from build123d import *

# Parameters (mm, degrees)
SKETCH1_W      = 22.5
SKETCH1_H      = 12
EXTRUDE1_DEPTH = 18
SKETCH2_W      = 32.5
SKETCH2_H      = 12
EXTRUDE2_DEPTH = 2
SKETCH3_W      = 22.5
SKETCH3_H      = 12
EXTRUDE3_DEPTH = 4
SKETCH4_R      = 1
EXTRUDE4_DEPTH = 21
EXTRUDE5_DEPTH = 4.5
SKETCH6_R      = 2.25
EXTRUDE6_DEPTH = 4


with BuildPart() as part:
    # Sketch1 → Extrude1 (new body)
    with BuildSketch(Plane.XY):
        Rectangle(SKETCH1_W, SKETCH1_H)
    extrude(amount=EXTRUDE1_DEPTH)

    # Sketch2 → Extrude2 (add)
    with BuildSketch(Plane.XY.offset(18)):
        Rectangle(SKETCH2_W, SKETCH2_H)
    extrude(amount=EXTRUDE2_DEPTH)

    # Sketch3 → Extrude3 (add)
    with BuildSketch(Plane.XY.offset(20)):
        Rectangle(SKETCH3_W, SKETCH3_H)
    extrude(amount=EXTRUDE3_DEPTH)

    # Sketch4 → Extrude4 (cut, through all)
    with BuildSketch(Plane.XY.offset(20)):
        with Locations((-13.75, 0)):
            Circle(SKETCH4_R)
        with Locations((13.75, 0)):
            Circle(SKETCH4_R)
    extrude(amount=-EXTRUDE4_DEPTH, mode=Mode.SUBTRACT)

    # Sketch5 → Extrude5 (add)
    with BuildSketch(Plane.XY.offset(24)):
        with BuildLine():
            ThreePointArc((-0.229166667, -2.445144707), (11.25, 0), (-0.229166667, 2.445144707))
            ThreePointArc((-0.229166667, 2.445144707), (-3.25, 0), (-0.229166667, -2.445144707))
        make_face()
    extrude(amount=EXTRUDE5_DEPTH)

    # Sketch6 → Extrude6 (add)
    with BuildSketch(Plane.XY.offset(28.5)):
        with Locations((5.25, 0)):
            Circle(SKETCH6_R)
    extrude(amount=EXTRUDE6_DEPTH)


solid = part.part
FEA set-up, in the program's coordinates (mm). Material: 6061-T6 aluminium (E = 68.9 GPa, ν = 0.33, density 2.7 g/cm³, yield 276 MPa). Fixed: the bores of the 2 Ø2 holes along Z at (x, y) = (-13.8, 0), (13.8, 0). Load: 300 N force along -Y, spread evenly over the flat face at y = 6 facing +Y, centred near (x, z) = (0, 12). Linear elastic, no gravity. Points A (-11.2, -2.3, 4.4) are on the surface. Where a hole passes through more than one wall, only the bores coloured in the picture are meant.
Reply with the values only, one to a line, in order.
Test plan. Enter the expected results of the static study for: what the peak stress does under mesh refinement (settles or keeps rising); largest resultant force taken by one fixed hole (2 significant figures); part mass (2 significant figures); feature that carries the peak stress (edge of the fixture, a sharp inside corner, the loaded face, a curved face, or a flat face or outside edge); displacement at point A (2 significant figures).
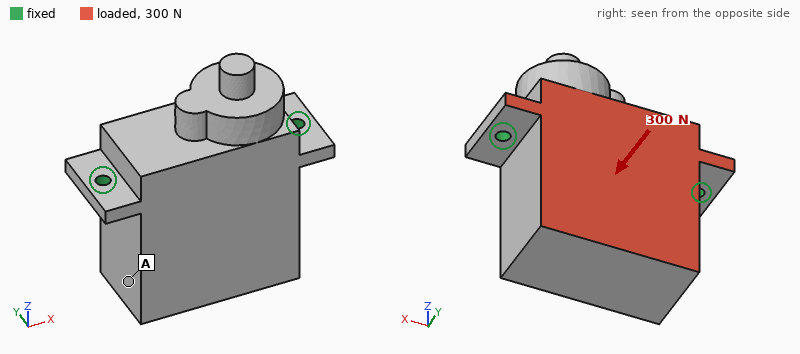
keeps rising
150 N
20 g
edge of the fixture
52 µm
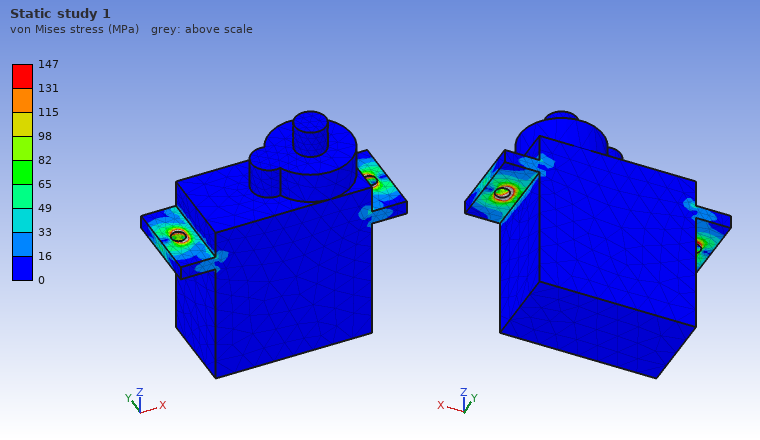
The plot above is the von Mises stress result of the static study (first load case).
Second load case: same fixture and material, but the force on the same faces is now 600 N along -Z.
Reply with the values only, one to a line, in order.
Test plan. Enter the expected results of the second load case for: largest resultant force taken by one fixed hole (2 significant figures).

300 N
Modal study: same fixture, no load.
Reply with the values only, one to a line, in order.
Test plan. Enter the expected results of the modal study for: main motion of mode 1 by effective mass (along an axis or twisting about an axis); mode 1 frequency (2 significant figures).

along Y
2700 Hz
